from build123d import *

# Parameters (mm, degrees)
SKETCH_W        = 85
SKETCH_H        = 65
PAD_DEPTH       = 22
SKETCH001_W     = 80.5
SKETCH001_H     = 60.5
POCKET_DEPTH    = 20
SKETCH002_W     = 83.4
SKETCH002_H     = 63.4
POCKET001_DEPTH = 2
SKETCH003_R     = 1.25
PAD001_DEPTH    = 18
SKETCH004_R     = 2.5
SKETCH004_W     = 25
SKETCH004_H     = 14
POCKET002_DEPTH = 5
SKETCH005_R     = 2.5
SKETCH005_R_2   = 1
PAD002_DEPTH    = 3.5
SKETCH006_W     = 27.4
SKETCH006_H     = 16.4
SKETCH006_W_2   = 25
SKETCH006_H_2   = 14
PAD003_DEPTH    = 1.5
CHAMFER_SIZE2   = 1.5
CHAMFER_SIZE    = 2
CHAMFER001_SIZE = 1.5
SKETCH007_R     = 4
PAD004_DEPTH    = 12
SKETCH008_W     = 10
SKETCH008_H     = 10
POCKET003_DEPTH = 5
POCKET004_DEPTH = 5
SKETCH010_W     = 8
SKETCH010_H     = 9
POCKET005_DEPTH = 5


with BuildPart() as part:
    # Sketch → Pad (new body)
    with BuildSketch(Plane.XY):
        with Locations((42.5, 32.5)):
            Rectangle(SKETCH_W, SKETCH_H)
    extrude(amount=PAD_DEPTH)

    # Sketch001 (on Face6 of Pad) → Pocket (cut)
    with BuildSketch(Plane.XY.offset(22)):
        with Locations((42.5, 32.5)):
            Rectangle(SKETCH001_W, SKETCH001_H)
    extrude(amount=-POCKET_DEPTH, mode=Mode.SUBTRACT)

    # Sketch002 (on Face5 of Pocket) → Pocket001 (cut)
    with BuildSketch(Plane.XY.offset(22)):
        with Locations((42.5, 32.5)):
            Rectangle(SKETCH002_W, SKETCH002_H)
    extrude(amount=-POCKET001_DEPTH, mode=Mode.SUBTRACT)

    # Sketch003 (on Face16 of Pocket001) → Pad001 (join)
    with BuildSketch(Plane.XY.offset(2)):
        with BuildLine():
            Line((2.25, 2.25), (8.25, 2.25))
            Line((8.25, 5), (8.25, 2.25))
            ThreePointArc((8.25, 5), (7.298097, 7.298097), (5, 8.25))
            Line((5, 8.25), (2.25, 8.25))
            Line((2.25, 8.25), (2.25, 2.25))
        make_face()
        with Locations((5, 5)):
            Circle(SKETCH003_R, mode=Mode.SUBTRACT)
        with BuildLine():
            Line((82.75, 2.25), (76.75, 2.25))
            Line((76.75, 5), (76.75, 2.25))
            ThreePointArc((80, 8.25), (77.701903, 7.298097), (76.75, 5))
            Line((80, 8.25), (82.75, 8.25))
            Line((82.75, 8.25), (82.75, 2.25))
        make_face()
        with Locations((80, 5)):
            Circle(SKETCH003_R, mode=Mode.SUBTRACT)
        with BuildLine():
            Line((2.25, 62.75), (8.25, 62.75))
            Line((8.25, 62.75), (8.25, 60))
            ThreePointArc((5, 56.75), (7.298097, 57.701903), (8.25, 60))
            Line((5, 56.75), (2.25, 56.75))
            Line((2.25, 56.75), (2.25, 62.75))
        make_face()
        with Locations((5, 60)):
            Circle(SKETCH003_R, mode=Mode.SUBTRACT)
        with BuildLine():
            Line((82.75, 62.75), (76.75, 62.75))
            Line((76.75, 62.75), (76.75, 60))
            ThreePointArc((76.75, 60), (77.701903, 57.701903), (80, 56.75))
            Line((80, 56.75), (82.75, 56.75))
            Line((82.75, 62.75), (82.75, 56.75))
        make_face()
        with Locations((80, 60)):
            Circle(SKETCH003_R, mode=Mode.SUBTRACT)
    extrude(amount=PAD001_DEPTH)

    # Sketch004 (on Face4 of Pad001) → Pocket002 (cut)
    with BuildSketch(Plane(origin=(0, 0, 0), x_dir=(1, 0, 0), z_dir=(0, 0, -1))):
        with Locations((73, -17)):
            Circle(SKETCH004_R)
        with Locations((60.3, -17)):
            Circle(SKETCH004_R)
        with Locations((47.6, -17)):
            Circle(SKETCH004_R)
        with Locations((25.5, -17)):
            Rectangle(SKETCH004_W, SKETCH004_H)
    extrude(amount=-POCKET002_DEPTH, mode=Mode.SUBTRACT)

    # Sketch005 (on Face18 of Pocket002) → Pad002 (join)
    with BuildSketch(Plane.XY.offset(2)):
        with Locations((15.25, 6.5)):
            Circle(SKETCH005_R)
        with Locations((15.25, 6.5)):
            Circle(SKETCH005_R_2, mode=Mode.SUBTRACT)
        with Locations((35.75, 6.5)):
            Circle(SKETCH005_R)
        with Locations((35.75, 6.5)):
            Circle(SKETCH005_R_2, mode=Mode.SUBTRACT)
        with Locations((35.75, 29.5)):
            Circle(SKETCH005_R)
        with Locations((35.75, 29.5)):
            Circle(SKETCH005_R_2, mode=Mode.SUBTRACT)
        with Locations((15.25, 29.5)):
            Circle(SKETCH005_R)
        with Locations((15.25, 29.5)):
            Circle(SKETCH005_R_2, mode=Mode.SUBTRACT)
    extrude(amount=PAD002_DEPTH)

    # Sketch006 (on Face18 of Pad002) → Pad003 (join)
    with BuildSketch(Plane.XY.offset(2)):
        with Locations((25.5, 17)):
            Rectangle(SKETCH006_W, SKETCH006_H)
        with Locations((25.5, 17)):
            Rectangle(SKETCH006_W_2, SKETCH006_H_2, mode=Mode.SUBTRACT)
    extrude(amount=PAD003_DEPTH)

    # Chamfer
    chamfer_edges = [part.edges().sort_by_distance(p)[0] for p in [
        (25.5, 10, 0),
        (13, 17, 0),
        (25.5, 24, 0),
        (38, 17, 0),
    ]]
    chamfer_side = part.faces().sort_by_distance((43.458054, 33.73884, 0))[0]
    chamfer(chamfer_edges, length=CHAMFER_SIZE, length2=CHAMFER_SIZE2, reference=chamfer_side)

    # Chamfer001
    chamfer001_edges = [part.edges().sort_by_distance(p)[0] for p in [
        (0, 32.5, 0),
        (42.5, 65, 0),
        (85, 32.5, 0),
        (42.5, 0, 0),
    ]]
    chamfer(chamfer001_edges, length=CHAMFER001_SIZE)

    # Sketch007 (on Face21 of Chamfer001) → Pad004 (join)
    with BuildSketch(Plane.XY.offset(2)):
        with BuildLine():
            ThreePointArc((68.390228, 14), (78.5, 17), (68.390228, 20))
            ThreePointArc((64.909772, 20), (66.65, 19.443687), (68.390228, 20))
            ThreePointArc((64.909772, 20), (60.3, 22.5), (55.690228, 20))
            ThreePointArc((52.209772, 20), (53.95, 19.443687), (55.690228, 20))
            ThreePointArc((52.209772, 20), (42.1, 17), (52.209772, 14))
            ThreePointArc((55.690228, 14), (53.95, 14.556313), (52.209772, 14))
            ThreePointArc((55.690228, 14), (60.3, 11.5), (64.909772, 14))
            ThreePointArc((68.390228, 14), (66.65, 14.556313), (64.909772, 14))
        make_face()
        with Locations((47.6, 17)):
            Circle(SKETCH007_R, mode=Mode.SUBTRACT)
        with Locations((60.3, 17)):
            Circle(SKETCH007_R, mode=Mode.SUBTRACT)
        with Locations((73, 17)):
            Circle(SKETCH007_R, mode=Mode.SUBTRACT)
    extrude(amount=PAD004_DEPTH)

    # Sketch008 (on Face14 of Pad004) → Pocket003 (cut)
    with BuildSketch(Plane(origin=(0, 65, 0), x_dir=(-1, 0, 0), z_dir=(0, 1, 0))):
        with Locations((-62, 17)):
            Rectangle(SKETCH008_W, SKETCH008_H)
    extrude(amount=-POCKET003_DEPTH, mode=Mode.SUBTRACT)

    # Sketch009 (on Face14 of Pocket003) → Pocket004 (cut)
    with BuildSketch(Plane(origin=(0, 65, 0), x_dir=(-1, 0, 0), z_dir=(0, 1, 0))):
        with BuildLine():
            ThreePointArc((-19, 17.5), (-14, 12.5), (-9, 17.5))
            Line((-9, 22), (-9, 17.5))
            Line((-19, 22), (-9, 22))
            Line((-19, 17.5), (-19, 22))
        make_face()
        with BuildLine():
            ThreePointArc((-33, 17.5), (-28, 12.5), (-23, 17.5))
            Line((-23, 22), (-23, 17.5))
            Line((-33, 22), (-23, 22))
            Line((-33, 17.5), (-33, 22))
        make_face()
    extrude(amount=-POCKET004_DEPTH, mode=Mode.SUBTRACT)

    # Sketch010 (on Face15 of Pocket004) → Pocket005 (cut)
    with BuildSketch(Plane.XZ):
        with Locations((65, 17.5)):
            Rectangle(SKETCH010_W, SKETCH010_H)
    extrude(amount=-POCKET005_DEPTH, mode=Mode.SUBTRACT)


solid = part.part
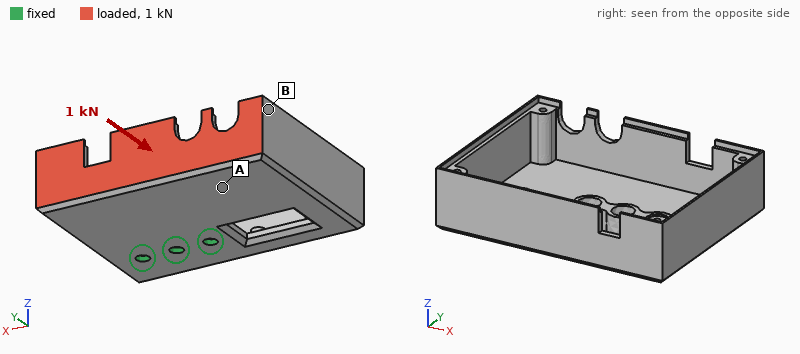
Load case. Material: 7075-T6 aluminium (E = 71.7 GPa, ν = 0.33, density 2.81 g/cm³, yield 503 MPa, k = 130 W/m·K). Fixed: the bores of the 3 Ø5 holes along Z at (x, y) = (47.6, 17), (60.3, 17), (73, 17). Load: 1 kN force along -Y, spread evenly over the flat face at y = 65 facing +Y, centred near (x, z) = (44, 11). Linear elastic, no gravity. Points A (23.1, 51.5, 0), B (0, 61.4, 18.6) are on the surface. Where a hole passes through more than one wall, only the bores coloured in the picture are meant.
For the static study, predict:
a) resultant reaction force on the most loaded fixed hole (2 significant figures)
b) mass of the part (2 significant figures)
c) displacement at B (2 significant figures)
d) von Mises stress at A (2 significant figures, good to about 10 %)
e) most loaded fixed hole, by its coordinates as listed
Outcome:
1.1 kN
72 g
1.2 mm
28 MPa
(47.6, 17)
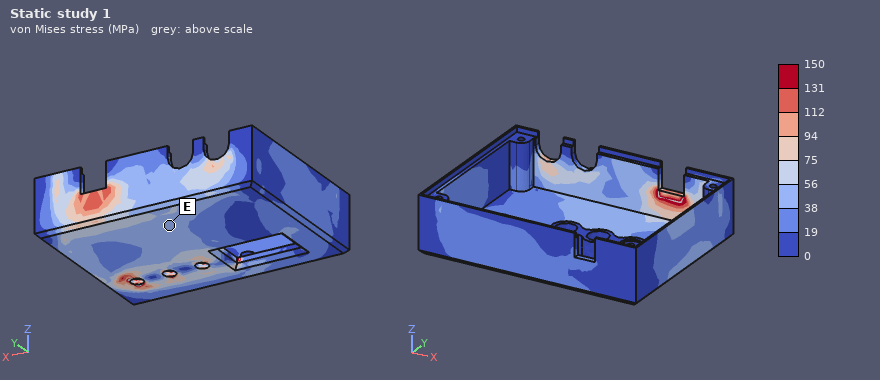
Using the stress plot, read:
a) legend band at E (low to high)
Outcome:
38 to 56 MPa
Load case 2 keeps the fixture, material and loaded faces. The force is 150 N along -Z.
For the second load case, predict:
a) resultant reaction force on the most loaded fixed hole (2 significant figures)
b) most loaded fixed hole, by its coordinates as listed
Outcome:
190 N
(47.6, 17)
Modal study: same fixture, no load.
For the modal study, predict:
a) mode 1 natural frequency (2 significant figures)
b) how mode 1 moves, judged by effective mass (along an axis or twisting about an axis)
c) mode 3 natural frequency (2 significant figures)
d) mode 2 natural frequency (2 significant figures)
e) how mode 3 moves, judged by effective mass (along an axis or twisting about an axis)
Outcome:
440 Hz
along Z
1100 Hz
1000 Hz
along Z
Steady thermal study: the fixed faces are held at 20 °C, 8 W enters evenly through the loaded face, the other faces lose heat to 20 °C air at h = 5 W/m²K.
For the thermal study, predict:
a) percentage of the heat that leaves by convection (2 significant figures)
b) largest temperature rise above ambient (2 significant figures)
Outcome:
12 %
19 K
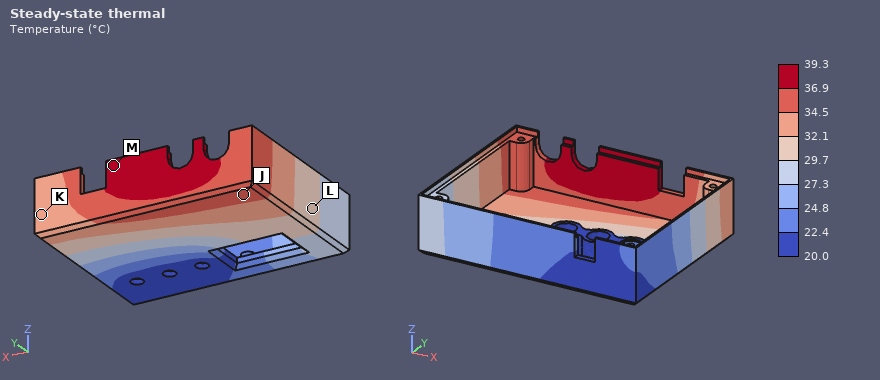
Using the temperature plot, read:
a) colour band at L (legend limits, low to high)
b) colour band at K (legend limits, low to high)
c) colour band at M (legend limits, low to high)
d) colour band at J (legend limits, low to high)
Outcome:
29.7 to 32.1 °C
32.1 to 34.5 °C
36.9 to 39.3 °C
34.5 to 36.9 °C
